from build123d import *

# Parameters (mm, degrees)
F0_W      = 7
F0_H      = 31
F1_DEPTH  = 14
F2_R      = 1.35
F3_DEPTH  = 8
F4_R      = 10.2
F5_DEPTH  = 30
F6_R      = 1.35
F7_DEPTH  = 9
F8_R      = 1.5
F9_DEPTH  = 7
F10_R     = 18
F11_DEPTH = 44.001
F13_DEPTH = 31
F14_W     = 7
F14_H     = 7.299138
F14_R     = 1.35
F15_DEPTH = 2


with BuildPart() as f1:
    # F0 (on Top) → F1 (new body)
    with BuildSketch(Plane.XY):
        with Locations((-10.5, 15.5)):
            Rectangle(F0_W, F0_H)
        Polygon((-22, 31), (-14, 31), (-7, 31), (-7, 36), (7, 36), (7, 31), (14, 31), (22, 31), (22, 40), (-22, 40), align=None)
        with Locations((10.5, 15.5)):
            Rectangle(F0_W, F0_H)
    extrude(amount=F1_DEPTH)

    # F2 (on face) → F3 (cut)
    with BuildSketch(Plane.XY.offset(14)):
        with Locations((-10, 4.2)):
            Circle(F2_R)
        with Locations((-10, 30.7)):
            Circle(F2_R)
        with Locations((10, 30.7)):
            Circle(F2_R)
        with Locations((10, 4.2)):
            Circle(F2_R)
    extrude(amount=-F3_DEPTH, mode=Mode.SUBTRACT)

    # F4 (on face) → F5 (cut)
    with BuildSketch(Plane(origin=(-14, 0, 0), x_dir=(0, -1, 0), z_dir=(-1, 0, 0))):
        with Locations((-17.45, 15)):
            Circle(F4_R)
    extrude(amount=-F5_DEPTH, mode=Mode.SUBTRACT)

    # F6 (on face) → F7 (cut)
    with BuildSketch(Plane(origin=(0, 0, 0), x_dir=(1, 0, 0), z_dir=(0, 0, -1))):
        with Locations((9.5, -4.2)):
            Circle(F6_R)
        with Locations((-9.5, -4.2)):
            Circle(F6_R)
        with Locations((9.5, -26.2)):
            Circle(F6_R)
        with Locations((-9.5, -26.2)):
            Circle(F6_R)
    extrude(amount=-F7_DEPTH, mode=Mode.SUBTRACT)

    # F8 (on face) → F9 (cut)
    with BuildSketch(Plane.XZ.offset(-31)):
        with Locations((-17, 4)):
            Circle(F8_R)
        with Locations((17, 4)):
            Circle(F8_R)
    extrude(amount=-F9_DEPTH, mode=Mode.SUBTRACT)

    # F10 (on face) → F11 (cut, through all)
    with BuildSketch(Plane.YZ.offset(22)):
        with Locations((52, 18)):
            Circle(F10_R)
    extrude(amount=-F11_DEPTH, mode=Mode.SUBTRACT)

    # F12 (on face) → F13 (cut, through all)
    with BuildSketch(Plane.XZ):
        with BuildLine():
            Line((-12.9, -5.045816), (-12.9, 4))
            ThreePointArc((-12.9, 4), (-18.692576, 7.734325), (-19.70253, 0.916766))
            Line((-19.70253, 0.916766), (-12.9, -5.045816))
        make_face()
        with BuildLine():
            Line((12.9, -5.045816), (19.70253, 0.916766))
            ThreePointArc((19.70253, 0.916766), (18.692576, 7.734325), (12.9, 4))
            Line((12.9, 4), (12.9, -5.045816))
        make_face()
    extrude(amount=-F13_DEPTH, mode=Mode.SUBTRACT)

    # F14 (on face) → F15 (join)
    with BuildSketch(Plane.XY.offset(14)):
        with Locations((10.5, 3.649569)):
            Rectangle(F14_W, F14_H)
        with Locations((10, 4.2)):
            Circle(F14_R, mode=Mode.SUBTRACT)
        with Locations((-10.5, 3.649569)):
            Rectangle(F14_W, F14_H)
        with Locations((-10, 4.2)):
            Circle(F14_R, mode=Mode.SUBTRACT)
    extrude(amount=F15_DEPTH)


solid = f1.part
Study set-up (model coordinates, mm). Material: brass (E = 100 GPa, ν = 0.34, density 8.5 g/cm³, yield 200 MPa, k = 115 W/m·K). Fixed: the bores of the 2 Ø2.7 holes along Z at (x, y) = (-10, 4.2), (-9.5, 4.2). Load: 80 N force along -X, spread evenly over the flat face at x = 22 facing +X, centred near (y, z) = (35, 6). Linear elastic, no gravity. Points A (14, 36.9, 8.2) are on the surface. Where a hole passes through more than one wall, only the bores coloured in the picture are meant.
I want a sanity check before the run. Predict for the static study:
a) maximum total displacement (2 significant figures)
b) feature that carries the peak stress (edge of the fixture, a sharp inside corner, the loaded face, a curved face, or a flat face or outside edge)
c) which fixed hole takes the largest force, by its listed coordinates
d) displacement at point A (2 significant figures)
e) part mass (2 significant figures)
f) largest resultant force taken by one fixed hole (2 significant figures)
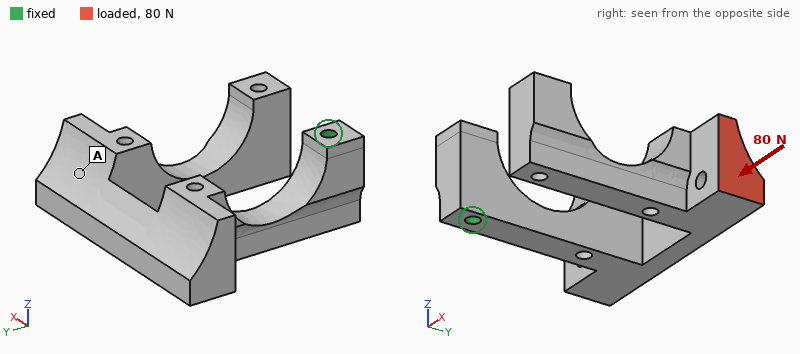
0.12 mm
edge of the fixture
(-9.5, 4.2)
0.11 mm
56 g
110 N
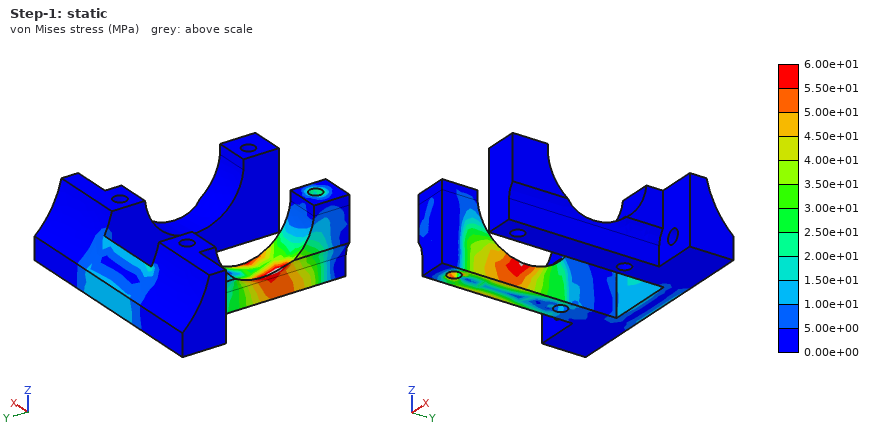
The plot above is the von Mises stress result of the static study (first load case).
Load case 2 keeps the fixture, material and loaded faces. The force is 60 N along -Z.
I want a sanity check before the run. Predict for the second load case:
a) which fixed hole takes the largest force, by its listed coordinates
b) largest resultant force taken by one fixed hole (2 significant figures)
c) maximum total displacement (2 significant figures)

(-9.5, 4.2)
92 N
0.33 mm
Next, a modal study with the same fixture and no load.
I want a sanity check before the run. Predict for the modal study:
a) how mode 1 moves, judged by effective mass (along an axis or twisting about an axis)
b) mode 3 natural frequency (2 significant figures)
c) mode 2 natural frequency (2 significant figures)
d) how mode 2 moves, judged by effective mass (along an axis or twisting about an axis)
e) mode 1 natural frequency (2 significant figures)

along Y
790 Hz
500 Hz
along Z
460 Hz
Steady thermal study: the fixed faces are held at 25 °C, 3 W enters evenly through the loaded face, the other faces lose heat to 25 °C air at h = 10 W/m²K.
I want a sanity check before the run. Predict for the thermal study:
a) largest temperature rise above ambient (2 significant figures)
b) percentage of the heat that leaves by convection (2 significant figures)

32 K
29 %
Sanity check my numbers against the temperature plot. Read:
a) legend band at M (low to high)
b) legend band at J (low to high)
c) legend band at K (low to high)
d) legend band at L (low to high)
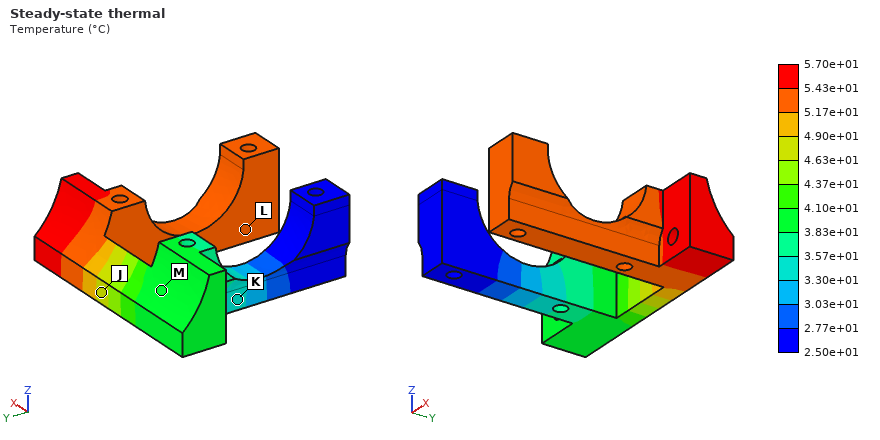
3.83e+01 to 4.10e+01 °C
4.63e+01 to 4.90e+01 °C
3.30e+01 to 3.57e+01 °C
5.17e+01 to 5.43e+01 °C
